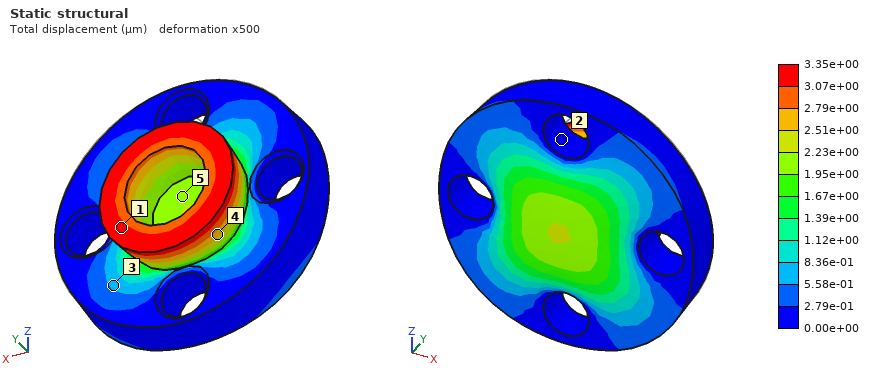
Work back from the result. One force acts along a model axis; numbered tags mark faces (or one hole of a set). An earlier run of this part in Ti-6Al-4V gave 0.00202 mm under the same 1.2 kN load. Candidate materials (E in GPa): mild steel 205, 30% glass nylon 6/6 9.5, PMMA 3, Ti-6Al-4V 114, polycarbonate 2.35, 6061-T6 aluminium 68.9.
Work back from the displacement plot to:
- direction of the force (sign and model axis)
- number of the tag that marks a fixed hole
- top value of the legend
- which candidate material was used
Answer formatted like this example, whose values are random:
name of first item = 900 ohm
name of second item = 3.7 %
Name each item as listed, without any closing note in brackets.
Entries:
direction of the force = -Y
number of the tag that marks a fixed hole = 2
top value of the legend = 3.35e+00 µm
which candidate material was used = 6061-T6 aluminium
